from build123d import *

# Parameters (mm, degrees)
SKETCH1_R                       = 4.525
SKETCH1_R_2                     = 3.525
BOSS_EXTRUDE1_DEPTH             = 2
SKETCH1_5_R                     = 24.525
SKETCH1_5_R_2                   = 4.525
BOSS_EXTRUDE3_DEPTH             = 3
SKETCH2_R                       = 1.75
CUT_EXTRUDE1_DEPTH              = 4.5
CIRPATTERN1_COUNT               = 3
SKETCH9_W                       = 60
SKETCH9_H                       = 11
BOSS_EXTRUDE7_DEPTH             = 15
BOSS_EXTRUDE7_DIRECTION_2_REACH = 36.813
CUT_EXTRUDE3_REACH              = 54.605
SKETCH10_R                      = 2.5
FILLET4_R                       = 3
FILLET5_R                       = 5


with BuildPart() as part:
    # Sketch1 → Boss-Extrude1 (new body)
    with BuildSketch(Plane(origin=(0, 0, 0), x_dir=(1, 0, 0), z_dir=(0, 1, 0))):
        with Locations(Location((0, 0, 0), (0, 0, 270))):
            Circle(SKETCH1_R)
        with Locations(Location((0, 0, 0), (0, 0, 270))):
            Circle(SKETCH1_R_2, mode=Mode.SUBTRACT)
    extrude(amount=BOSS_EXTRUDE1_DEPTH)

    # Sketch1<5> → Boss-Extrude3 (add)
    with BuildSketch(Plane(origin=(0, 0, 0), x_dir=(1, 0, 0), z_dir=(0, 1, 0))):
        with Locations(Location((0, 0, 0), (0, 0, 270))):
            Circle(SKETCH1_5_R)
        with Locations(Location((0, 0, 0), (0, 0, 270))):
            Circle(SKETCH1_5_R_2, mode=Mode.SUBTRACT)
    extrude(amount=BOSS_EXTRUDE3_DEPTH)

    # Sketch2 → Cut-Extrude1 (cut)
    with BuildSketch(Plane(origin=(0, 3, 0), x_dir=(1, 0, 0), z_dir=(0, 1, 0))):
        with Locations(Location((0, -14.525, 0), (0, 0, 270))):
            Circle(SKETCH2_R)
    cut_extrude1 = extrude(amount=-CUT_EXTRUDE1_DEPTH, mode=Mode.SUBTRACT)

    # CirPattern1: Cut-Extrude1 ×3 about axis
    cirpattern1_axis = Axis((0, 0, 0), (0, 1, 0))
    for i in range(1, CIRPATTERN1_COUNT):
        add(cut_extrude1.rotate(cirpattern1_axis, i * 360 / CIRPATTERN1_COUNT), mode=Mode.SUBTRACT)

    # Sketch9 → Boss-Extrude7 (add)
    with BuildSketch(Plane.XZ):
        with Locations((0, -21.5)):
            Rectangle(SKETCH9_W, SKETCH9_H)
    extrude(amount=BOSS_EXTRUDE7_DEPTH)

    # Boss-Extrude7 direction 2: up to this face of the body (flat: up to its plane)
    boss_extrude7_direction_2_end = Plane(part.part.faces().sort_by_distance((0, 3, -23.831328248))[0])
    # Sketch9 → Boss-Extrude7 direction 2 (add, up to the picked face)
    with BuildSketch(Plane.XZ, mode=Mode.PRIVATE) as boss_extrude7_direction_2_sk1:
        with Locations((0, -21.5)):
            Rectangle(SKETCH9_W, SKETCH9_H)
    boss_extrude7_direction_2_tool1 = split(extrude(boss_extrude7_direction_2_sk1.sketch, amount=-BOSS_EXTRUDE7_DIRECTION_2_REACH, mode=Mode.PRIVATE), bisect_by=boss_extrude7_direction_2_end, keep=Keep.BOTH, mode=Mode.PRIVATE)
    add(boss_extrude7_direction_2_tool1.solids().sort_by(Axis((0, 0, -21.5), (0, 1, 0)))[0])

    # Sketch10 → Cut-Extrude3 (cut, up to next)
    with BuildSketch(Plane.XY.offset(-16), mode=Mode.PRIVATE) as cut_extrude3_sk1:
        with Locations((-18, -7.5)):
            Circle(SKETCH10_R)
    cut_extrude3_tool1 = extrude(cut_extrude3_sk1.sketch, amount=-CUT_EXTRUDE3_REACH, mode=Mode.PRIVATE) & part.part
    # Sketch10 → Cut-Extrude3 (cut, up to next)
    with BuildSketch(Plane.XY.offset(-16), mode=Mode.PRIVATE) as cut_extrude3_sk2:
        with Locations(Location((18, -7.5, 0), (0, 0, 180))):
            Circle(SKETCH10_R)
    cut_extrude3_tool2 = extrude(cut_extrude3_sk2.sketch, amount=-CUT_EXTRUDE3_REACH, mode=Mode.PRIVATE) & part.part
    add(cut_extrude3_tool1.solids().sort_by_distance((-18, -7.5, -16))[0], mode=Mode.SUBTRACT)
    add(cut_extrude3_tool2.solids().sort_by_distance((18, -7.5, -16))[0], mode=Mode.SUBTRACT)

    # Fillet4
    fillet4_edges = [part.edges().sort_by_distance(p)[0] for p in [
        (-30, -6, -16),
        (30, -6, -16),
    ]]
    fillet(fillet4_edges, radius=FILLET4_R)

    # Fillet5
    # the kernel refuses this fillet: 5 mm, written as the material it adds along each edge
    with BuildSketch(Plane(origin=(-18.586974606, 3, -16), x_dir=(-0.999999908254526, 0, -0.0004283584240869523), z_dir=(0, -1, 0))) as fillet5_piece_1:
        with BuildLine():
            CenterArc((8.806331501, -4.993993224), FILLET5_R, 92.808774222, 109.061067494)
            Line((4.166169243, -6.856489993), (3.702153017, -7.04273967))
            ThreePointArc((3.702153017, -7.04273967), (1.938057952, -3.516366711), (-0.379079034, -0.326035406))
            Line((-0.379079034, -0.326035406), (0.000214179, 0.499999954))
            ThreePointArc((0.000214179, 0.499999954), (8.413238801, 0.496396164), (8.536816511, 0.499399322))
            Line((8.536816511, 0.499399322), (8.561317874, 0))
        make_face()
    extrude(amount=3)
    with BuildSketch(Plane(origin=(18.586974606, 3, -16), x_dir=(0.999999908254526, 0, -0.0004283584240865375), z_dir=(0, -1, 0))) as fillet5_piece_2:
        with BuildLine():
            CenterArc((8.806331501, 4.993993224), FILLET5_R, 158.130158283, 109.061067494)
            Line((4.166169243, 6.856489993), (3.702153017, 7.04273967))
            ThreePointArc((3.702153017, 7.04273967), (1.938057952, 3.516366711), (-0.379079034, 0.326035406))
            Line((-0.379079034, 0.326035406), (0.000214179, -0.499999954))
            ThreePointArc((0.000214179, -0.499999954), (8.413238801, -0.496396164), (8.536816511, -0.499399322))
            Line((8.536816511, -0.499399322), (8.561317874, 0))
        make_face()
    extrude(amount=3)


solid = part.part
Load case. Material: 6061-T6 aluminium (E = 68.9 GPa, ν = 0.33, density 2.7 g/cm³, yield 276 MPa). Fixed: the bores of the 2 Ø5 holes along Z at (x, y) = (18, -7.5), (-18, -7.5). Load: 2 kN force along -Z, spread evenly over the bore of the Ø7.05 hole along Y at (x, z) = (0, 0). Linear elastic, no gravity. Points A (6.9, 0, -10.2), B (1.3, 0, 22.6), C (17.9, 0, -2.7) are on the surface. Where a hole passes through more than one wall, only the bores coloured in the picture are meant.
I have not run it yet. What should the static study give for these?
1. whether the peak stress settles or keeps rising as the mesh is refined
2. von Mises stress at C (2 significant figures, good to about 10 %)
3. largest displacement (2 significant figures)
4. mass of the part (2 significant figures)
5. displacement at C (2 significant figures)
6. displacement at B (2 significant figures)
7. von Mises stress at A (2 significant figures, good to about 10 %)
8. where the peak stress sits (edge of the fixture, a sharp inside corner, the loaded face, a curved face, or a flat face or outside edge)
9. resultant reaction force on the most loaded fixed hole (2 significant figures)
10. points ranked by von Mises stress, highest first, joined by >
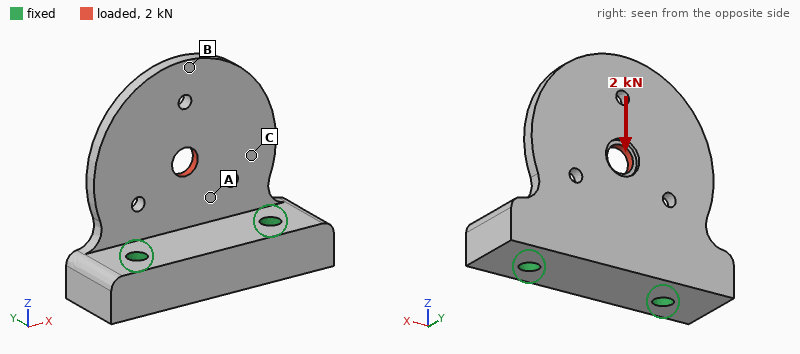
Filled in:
keeps rising
19 MPa
58 µm
44 g
9.2 µm
54 µm
32 MPa
a sharp inside corner
1.0 kN
A > C > B
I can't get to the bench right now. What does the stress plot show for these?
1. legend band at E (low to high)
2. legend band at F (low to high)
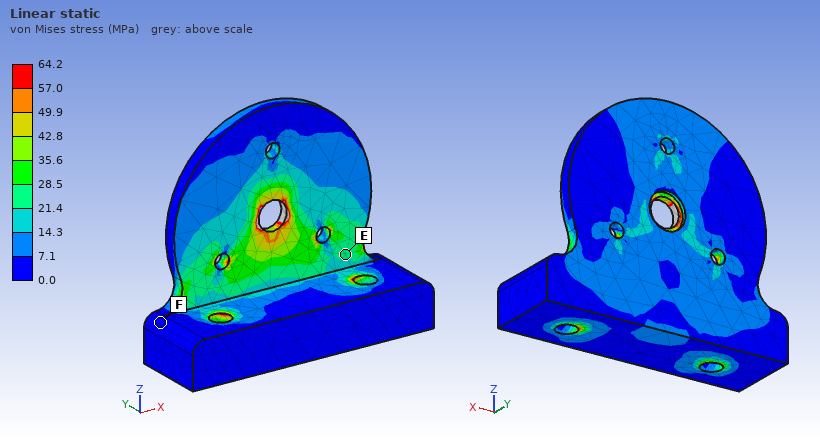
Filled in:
21.4 to 28.5 MPa
0.0 to 7.1 MPa
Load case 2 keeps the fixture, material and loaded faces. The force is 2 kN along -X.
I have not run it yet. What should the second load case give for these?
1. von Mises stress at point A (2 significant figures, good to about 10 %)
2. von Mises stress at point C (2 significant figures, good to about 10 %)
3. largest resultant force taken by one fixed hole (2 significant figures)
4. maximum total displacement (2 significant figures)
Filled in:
36 MPa
19 MPa
1.5 kN
37 µm
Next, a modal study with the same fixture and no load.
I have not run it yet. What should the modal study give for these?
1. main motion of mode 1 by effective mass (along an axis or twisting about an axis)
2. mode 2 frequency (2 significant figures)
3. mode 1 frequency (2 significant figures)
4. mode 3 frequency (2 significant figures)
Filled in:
along Y
4000 Hz
1600 Hz
8300 Hz
